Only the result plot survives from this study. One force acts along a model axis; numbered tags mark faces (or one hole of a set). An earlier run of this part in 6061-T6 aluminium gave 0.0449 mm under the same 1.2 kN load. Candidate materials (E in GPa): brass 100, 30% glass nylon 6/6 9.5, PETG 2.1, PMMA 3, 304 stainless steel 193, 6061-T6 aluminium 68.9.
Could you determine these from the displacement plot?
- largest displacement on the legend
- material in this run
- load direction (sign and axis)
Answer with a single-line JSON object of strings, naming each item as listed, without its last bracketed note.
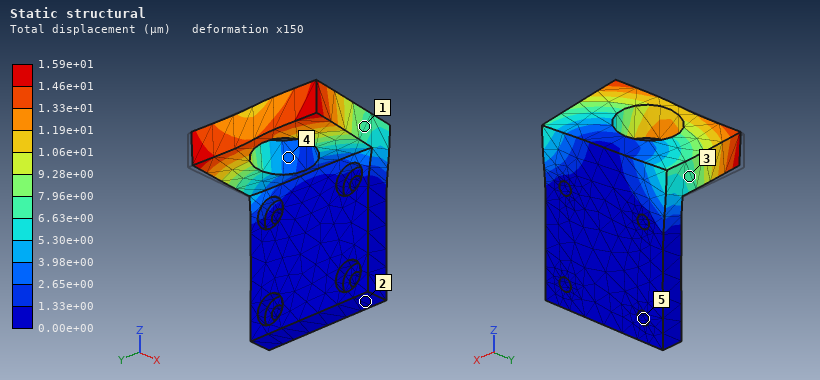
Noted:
{"largest displacement on the legend": "1.59e+01 µm", "material in this run": "304 stainless steel", "load direction": "-Y"}
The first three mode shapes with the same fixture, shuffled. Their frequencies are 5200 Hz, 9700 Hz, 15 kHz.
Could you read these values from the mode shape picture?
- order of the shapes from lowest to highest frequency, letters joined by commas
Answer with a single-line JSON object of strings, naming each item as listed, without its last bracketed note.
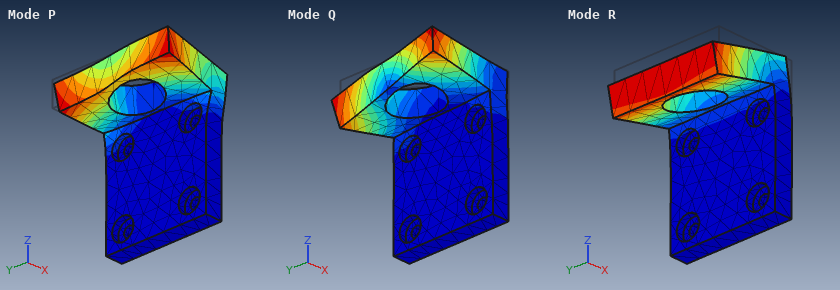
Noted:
{"order of the shapes from lowest to highest frequency, letters joined by commas": "R, P, Q"}
